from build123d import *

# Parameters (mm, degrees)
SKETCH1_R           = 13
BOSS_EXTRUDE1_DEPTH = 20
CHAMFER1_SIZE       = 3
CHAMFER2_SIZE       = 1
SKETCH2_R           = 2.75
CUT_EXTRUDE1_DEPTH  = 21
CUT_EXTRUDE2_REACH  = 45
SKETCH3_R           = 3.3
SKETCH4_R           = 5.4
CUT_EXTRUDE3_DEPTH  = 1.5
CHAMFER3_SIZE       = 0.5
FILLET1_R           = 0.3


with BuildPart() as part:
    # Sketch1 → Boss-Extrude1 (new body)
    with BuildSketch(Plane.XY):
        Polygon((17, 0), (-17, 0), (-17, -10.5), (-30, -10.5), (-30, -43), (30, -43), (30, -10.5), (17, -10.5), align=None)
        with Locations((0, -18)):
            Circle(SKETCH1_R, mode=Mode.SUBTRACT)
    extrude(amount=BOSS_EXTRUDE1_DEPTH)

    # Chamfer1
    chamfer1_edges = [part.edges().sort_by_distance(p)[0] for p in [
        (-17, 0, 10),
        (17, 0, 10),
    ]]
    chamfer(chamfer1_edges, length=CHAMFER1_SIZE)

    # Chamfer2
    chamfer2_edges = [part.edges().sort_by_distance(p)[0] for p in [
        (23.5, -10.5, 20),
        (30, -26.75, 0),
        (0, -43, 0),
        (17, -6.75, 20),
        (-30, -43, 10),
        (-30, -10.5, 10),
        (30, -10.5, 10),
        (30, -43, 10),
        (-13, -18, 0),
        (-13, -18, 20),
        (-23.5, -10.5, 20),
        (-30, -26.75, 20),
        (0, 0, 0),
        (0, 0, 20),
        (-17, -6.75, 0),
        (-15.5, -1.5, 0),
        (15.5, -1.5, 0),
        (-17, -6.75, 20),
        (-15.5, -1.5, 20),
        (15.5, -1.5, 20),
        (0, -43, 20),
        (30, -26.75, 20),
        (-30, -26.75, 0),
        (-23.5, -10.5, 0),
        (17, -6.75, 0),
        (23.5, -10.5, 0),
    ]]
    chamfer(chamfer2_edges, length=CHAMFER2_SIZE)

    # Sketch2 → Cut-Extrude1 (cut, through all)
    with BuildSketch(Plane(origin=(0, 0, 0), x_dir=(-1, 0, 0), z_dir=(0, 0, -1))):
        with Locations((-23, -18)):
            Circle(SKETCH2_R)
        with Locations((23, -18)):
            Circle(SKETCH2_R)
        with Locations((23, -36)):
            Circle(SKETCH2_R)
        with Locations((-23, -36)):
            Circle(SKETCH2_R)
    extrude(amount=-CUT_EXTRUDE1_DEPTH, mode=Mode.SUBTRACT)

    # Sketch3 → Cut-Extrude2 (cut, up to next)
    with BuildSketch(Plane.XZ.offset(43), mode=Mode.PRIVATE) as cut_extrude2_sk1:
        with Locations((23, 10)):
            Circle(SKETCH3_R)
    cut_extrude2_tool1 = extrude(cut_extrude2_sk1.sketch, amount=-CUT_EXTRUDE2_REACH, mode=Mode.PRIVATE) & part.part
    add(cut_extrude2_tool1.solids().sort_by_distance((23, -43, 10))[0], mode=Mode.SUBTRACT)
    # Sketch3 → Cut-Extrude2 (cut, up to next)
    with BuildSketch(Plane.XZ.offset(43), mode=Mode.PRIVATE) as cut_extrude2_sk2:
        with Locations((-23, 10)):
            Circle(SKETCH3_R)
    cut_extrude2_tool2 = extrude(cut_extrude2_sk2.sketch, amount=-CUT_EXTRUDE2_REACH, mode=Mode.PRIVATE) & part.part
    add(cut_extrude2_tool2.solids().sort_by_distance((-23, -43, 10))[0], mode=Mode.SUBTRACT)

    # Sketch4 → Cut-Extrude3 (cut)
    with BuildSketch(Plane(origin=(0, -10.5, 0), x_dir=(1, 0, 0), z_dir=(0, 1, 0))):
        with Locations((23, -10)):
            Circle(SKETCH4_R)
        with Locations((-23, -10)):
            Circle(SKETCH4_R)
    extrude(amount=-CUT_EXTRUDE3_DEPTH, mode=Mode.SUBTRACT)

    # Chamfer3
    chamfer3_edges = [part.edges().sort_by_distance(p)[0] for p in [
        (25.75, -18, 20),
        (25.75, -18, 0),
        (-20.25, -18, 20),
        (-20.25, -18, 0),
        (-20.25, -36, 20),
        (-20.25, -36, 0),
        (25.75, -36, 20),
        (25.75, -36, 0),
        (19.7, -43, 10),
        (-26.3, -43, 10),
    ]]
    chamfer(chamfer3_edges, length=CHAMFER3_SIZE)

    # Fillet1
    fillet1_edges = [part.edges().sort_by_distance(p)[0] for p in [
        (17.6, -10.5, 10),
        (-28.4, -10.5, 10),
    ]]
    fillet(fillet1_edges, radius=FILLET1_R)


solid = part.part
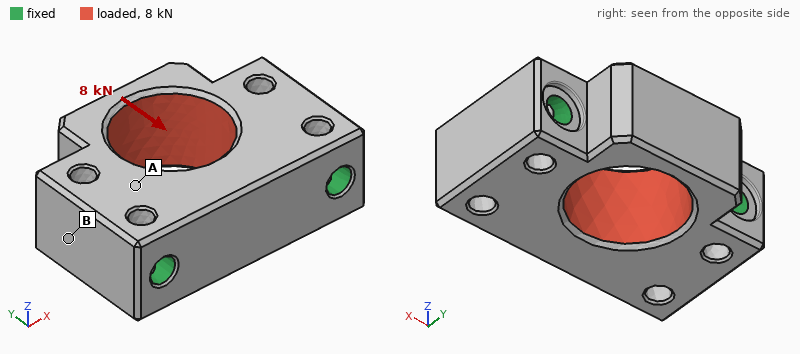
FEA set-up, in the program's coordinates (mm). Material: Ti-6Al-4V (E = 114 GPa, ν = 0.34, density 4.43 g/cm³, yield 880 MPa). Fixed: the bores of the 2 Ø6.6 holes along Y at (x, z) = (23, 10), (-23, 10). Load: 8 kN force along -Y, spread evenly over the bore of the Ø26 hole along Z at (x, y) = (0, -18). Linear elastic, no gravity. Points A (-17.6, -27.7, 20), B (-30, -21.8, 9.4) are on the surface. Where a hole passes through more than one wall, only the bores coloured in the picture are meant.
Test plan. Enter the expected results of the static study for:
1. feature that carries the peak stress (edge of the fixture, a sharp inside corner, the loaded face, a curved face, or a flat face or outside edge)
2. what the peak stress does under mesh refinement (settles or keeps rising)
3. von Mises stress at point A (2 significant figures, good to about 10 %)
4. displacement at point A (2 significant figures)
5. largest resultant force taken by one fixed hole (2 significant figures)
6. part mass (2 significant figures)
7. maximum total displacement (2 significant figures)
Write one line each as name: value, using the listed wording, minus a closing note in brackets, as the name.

feature that carries the peak stress: edge of the fixture
what the peak stress does under mesh refinement: keeps rising
von Mises stress at point A: 7.9 MPa
displacement at point A: 0.94 µm
largest resultant force taken by one fixed hole: 4.1 kN
part mass: 140 g
maximum total displacement: 5.9 µm
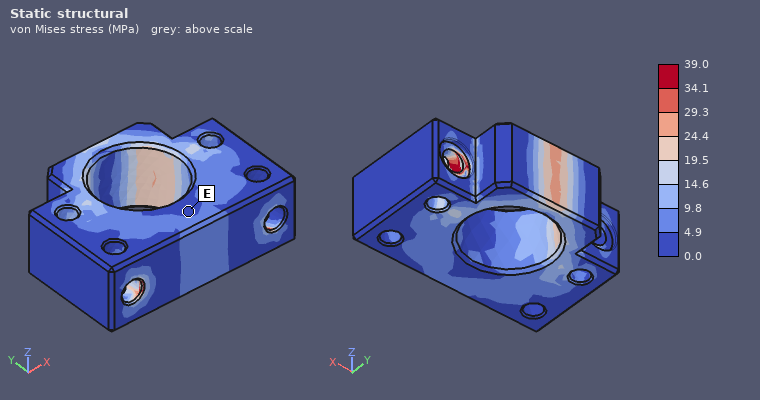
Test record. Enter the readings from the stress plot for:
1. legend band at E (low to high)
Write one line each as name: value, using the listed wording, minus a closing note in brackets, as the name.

legend band at E: 0.0 to 4.9 MPa
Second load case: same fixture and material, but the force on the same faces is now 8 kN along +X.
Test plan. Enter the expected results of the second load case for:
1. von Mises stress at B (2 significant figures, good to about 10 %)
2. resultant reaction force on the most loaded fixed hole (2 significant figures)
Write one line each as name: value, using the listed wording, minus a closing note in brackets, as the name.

von Mises stress at B: 4.9 MPa
resultant reaction force on the most loaded fixed hole: 4.0 kN
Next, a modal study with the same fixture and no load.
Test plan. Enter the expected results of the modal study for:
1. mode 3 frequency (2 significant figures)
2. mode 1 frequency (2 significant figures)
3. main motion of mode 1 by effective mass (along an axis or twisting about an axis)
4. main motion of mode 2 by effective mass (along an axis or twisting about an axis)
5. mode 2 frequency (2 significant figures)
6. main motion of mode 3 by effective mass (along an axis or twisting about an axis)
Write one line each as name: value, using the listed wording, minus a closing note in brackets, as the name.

mode 3 frequency: 26 kHz
mode 1 frequency: 16 kHz
main motion of mode 1 by effective mass: along Z
main motion of mode 2 by effective mass: along X
mode 2 frequency: 23 kHz
main motion of mode 3 by effective mass: along Z
